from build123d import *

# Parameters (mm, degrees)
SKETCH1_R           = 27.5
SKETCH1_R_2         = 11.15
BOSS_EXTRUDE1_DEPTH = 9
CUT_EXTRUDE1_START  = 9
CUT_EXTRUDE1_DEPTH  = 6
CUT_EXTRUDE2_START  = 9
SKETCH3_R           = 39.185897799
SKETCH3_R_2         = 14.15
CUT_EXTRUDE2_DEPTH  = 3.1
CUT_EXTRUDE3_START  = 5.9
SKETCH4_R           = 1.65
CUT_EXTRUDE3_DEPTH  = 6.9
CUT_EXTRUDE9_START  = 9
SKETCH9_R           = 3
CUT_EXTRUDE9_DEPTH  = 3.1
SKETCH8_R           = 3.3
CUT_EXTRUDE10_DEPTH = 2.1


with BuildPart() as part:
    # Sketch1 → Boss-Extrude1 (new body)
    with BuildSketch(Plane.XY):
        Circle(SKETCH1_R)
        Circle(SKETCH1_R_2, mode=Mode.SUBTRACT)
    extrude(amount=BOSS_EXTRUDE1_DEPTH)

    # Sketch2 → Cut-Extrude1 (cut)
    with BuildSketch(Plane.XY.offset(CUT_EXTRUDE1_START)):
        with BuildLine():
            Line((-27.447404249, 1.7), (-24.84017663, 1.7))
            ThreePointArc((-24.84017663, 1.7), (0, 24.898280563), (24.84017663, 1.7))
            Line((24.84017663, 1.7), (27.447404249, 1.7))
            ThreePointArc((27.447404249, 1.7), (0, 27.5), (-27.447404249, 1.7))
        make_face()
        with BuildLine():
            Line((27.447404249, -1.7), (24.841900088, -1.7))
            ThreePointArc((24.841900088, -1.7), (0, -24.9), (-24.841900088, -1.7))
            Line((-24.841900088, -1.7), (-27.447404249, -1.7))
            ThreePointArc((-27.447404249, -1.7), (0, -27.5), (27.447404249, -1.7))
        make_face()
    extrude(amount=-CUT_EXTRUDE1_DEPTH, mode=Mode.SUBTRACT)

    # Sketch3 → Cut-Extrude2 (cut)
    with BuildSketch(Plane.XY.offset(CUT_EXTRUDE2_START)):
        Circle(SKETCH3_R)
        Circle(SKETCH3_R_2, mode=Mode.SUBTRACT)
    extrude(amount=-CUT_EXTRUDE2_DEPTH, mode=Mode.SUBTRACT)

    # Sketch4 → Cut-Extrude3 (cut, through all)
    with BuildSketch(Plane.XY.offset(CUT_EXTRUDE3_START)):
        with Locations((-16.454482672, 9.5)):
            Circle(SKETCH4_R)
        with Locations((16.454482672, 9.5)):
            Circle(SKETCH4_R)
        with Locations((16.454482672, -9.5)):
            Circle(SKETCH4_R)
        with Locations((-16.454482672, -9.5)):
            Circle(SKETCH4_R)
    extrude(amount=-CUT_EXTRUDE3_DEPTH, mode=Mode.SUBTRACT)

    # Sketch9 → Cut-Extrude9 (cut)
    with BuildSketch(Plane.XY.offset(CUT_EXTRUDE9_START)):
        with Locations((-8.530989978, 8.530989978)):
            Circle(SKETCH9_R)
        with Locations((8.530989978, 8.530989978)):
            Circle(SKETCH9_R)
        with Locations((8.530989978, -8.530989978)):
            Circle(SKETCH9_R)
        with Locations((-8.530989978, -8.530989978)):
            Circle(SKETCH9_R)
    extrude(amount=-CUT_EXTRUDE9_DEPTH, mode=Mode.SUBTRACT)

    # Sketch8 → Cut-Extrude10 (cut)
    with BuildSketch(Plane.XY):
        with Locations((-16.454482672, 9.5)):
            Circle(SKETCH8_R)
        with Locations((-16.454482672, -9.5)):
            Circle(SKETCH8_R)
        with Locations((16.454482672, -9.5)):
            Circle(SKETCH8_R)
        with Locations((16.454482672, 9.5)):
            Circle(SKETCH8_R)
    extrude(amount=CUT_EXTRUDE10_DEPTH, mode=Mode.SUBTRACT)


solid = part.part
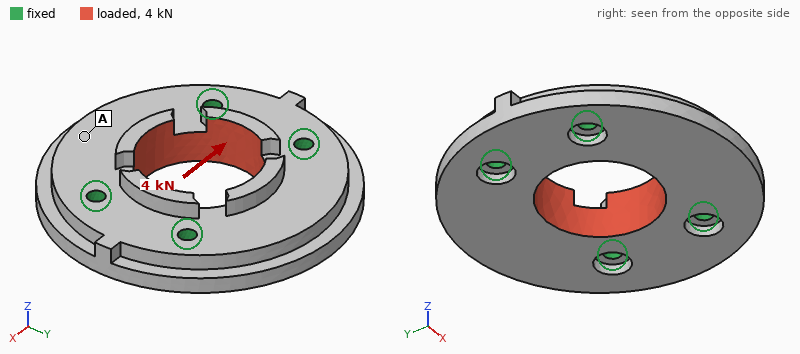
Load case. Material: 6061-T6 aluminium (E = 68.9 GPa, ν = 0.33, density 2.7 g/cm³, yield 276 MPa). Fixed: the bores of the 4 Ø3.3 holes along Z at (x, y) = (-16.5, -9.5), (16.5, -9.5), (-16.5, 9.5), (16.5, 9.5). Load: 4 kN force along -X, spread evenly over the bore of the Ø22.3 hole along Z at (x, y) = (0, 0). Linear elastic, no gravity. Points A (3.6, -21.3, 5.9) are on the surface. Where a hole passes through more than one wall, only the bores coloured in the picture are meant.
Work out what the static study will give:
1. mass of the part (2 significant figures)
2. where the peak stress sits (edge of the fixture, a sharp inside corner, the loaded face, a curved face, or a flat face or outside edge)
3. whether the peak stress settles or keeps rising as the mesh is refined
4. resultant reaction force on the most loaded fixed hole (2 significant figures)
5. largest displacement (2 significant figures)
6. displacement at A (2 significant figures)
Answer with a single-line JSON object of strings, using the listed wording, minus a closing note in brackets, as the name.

{"mass of the part": "29 g", "where the peak stress sits": "edge of the fixture", "whether the peak stress settles or keeps rising as the mesh is refined": "keeps rising", "resultant reaction force on the most loaded fixed hole": "1.0 kN", "largest displacement": "5.2 µm", "displacement at A": "1.9 µm"}
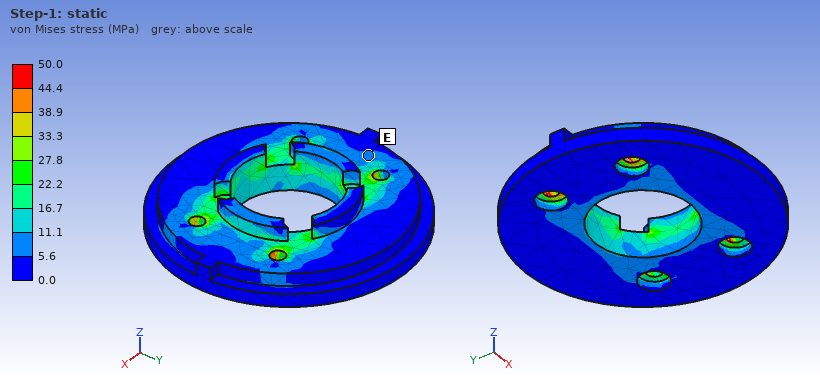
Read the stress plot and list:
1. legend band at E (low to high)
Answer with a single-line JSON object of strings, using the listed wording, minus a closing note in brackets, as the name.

{"legend band at E": "5.6 to 11.1 MPa"}
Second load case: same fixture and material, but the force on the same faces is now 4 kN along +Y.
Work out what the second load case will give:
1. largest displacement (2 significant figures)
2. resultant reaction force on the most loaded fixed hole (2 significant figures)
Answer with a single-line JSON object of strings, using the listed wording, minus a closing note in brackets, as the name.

{"largest displacement": "9.2 µm", "resultant reaction force on the most loaded fixed hole": "1.0 kN"}
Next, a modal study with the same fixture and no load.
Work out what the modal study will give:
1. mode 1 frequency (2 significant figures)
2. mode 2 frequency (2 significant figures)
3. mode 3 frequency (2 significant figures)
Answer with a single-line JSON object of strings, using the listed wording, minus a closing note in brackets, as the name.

{"mode 1 frequency": "11 kHz", "mode 2 frequency": "11 kHz", "mode 3 frequency": "25 kHz"}
